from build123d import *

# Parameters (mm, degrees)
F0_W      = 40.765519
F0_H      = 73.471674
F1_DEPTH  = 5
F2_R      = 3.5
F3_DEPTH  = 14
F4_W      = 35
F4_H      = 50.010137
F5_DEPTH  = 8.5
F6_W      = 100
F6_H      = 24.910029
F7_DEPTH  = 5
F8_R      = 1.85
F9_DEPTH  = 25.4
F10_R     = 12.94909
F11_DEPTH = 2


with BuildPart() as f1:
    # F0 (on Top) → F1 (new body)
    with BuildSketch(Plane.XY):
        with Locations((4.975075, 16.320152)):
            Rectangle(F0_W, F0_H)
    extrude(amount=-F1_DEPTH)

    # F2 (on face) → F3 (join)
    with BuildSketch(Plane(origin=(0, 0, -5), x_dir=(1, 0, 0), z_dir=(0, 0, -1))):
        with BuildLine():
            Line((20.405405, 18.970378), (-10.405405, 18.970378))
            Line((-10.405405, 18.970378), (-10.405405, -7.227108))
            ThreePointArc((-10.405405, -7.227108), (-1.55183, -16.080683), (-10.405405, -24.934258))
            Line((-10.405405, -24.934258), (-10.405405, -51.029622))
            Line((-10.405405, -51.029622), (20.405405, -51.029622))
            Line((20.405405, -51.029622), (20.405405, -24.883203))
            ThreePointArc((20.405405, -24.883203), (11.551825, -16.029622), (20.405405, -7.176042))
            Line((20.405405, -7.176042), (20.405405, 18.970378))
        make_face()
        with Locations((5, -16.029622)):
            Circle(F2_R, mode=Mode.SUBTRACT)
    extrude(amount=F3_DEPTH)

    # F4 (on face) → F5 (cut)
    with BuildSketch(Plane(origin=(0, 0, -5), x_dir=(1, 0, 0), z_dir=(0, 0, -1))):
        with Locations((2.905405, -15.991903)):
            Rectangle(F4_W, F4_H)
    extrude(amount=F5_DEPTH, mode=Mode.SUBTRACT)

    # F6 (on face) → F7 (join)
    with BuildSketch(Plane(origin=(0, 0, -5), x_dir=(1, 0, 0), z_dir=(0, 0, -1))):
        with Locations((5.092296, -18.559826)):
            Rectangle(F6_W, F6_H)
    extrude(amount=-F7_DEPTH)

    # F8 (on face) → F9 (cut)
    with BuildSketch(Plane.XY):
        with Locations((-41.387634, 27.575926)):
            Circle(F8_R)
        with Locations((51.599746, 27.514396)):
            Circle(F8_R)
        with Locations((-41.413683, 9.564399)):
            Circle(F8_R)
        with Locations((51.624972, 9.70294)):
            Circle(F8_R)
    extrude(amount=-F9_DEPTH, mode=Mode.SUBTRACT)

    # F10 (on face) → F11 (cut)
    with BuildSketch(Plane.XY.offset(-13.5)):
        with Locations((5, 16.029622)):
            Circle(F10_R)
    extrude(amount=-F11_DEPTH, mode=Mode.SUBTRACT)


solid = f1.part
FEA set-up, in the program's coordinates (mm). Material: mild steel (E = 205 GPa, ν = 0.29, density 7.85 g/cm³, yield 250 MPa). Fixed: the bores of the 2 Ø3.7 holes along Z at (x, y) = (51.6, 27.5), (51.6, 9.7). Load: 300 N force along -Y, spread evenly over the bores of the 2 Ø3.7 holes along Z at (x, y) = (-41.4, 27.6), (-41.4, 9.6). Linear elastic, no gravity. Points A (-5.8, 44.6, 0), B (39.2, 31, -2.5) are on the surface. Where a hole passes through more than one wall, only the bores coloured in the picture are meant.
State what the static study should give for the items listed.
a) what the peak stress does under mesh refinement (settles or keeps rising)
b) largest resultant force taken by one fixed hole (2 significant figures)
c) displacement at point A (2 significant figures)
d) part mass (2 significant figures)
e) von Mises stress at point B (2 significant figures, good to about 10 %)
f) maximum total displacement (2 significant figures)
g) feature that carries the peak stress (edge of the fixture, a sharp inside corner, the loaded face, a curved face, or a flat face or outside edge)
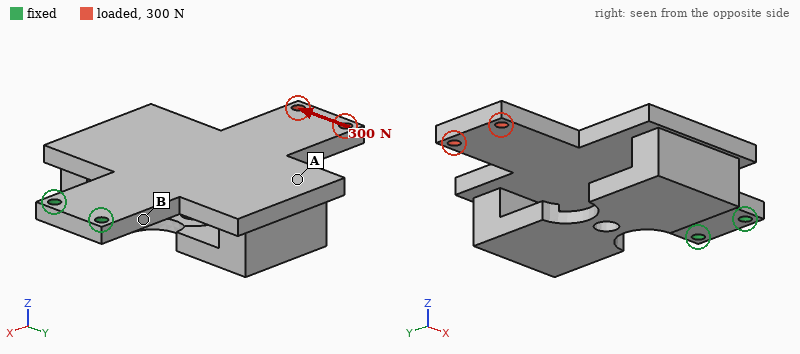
keeps rising
1.5 kN
30 µm
290 g
47 MPa
54 µm
edge of the fixture
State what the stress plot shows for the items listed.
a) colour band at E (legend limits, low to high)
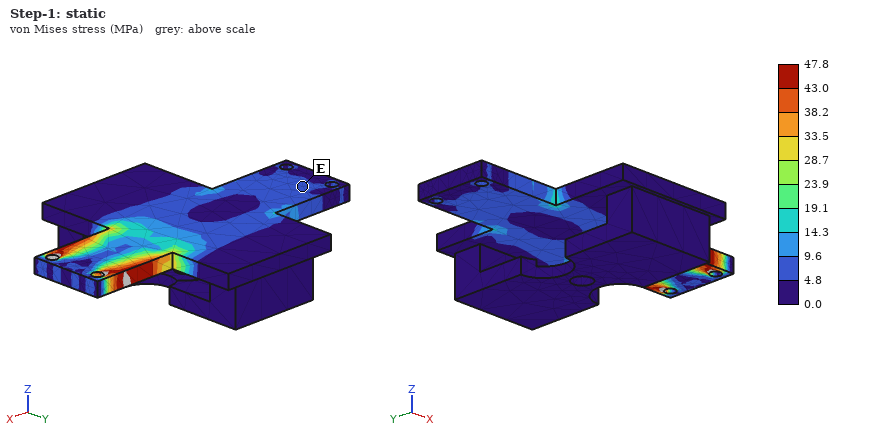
4.8 to 9.6 MPa
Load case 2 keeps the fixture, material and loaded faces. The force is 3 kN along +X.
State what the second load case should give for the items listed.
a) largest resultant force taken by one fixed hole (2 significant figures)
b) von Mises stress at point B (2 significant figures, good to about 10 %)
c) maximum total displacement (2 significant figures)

1.5 kN
26 MPa
12 µm
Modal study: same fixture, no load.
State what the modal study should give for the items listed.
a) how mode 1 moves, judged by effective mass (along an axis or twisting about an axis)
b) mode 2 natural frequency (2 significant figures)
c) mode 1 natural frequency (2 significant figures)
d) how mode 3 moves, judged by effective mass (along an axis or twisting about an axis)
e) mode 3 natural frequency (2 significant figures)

along Z
690 Hz
320 Hz
along Y
1400 Hz
